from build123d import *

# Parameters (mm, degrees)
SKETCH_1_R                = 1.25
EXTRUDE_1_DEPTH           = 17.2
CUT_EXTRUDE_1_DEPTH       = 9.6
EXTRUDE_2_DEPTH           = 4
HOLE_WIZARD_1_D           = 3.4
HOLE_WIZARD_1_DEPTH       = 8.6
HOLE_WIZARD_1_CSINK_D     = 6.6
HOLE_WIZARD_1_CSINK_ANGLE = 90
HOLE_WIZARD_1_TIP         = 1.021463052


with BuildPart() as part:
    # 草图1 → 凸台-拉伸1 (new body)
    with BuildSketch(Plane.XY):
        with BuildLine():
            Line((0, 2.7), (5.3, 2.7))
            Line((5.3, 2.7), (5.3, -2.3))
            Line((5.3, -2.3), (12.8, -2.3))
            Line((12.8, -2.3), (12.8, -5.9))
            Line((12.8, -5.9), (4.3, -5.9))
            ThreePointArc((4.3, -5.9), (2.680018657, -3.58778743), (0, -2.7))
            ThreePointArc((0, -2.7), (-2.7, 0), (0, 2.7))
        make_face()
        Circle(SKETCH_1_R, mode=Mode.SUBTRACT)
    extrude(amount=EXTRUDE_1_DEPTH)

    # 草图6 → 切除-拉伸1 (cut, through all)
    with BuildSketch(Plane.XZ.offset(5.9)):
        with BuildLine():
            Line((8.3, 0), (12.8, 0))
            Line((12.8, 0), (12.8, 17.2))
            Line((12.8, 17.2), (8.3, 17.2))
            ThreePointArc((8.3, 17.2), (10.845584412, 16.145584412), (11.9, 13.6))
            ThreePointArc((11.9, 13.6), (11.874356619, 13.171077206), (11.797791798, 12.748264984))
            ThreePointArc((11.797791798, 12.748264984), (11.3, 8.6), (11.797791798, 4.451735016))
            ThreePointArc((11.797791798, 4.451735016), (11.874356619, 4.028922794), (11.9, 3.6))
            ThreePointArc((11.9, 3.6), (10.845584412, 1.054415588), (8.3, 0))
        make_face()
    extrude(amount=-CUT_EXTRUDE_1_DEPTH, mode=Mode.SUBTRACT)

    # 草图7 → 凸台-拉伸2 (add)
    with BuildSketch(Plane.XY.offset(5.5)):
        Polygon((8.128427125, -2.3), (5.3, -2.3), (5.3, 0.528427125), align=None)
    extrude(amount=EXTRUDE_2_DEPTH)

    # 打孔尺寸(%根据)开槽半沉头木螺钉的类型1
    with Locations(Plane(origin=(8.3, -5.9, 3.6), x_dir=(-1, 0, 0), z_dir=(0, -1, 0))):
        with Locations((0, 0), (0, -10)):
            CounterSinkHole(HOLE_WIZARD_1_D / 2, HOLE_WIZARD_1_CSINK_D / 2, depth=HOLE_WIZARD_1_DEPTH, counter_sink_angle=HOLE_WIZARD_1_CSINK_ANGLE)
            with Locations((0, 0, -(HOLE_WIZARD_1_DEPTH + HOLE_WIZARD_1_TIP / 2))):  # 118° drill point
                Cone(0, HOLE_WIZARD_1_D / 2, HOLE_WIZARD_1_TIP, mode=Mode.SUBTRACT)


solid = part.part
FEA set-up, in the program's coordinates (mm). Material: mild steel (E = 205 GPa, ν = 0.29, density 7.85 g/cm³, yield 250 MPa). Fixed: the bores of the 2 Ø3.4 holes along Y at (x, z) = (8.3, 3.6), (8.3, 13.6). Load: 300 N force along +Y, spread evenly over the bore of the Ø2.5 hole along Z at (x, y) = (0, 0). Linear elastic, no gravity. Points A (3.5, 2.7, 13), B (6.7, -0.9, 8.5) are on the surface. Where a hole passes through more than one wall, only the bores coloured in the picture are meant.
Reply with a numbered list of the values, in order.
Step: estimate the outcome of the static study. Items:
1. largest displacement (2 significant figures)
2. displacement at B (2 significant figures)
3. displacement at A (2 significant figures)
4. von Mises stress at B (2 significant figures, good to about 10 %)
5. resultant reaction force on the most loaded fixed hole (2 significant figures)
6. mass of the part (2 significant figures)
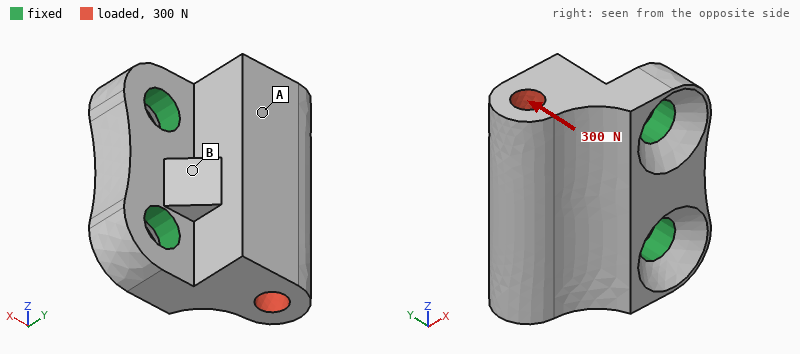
1. 9.7 µm
2. 2.0 µm
3. 6.4 µm
4. 46 MPa
5. 160 N
6. 7.9 g
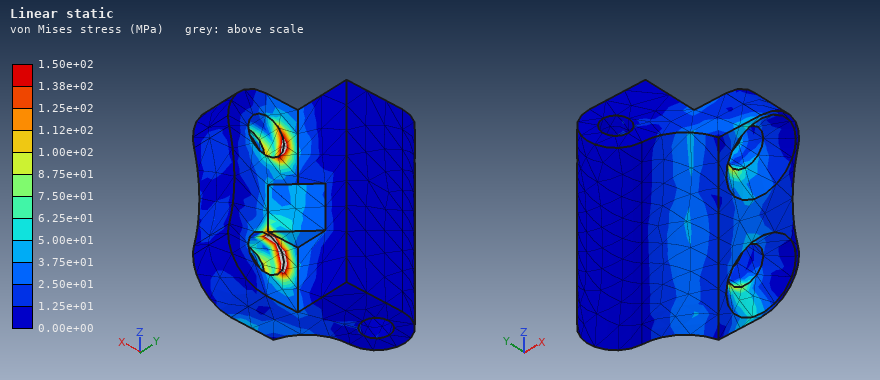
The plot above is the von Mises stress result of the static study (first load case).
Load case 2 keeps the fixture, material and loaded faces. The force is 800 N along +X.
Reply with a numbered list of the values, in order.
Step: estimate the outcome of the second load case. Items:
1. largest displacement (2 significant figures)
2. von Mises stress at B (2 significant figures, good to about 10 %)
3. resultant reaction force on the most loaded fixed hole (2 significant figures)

1. 13 µm
2. 81 MPa
3. 420 N
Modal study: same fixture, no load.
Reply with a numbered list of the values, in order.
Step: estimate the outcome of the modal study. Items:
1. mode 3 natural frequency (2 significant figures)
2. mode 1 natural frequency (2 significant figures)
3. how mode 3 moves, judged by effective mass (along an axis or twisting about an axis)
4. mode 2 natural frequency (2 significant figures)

1. 43 kHz
2. 16 kHz
3. along Z
4. 35 kHz
